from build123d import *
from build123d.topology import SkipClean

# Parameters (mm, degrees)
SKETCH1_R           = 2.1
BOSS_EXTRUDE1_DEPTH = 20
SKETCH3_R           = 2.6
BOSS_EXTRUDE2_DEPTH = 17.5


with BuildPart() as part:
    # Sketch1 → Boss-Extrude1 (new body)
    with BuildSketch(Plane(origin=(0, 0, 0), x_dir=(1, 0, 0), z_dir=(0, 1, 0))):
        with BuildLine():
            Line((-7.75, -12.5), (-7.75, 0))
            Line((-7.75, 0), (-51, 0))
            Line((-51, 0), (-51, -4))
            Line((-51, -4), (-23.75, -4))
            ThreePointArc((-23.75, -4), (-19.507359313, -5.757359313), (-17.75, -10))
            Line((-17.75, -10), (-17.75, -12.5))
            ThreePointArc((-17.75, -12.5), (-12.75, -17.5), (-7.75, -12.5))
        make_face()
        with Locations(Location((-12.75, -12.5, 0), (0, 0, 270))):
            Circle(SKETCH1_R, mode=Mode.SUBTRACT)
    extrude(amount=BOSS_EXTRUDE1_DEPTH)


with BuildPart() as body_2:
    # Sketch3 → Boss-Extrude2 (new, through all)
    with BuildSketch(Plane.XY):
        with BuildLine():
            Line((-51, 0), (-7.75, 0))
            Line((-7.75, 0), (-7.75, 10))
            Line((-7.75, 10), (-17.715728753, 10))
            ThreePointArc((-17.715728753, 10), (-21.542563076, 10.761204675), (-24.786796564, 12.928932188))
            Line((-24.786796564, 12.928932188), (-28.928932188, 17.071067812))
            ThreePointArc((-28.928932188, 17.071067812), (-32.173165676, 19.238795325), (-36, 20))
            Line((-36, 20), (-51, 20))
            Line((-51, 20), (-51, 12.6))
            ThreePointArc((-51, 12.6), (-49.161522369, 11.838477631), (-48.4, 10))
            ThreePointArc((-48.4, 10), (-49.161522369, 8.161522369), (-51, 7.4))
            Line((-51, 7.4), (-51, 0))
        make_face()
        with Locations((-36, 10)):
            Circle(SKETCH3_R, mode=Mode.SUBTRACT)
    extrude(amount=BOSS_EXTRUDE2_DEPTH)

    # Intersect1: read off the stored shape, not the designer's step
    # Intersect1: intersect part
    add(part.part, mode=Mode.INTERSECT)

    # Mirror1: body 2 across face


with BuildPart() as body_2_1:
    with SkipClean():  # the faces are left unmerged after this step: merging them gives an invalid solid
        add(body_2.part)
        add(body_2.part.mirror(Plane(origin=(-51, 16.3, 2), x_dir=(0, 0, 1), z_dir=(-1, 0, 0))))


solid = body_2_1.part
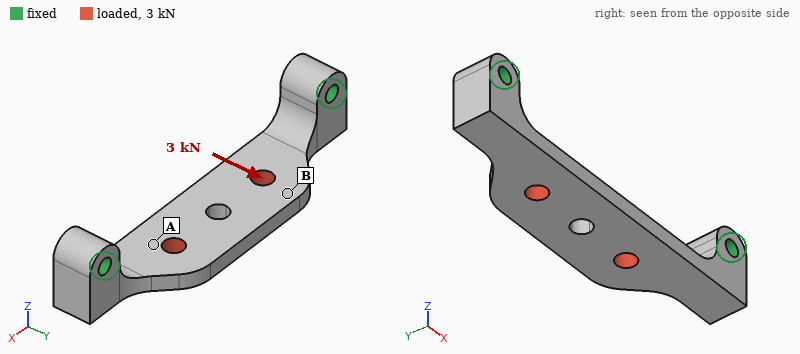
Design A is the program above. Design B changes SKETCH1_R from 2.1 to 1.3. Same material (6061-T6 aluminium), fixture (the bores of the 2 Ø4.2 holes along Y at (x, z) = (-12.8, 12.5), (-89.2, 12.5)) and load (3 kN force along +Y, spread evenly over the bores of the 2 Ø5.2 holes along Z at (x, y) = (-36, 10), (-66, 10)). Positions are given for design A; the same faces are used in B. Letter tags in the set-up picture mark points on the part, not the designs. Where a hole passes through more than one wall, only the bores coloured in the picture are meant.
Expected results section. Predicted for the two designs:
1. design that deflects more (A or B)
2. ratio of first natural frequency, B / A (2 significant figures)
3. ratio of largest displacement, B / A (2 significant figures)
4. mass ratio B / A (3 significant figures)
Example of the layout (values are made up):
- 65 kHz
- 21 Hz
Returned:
- B
- 1.00
- 1.1
- 1.02
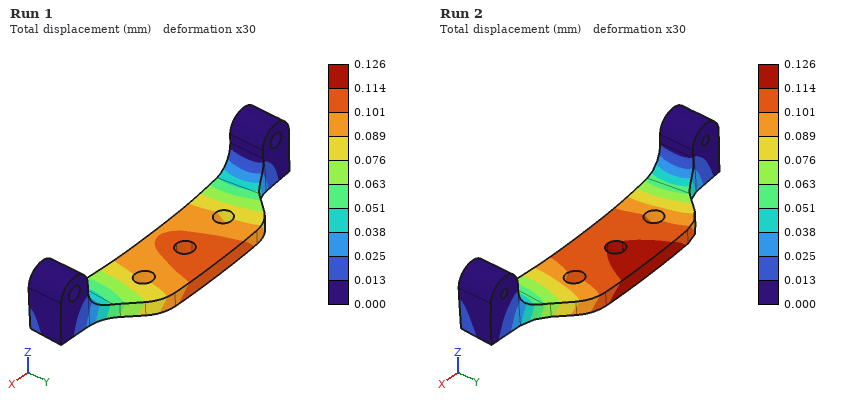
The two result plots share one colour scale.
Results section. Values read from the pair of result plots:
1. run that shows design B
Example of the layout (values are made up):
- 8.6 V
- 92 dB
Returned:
- Run 2
